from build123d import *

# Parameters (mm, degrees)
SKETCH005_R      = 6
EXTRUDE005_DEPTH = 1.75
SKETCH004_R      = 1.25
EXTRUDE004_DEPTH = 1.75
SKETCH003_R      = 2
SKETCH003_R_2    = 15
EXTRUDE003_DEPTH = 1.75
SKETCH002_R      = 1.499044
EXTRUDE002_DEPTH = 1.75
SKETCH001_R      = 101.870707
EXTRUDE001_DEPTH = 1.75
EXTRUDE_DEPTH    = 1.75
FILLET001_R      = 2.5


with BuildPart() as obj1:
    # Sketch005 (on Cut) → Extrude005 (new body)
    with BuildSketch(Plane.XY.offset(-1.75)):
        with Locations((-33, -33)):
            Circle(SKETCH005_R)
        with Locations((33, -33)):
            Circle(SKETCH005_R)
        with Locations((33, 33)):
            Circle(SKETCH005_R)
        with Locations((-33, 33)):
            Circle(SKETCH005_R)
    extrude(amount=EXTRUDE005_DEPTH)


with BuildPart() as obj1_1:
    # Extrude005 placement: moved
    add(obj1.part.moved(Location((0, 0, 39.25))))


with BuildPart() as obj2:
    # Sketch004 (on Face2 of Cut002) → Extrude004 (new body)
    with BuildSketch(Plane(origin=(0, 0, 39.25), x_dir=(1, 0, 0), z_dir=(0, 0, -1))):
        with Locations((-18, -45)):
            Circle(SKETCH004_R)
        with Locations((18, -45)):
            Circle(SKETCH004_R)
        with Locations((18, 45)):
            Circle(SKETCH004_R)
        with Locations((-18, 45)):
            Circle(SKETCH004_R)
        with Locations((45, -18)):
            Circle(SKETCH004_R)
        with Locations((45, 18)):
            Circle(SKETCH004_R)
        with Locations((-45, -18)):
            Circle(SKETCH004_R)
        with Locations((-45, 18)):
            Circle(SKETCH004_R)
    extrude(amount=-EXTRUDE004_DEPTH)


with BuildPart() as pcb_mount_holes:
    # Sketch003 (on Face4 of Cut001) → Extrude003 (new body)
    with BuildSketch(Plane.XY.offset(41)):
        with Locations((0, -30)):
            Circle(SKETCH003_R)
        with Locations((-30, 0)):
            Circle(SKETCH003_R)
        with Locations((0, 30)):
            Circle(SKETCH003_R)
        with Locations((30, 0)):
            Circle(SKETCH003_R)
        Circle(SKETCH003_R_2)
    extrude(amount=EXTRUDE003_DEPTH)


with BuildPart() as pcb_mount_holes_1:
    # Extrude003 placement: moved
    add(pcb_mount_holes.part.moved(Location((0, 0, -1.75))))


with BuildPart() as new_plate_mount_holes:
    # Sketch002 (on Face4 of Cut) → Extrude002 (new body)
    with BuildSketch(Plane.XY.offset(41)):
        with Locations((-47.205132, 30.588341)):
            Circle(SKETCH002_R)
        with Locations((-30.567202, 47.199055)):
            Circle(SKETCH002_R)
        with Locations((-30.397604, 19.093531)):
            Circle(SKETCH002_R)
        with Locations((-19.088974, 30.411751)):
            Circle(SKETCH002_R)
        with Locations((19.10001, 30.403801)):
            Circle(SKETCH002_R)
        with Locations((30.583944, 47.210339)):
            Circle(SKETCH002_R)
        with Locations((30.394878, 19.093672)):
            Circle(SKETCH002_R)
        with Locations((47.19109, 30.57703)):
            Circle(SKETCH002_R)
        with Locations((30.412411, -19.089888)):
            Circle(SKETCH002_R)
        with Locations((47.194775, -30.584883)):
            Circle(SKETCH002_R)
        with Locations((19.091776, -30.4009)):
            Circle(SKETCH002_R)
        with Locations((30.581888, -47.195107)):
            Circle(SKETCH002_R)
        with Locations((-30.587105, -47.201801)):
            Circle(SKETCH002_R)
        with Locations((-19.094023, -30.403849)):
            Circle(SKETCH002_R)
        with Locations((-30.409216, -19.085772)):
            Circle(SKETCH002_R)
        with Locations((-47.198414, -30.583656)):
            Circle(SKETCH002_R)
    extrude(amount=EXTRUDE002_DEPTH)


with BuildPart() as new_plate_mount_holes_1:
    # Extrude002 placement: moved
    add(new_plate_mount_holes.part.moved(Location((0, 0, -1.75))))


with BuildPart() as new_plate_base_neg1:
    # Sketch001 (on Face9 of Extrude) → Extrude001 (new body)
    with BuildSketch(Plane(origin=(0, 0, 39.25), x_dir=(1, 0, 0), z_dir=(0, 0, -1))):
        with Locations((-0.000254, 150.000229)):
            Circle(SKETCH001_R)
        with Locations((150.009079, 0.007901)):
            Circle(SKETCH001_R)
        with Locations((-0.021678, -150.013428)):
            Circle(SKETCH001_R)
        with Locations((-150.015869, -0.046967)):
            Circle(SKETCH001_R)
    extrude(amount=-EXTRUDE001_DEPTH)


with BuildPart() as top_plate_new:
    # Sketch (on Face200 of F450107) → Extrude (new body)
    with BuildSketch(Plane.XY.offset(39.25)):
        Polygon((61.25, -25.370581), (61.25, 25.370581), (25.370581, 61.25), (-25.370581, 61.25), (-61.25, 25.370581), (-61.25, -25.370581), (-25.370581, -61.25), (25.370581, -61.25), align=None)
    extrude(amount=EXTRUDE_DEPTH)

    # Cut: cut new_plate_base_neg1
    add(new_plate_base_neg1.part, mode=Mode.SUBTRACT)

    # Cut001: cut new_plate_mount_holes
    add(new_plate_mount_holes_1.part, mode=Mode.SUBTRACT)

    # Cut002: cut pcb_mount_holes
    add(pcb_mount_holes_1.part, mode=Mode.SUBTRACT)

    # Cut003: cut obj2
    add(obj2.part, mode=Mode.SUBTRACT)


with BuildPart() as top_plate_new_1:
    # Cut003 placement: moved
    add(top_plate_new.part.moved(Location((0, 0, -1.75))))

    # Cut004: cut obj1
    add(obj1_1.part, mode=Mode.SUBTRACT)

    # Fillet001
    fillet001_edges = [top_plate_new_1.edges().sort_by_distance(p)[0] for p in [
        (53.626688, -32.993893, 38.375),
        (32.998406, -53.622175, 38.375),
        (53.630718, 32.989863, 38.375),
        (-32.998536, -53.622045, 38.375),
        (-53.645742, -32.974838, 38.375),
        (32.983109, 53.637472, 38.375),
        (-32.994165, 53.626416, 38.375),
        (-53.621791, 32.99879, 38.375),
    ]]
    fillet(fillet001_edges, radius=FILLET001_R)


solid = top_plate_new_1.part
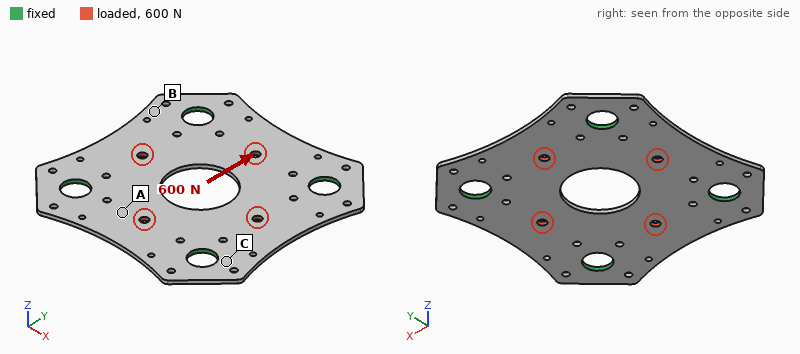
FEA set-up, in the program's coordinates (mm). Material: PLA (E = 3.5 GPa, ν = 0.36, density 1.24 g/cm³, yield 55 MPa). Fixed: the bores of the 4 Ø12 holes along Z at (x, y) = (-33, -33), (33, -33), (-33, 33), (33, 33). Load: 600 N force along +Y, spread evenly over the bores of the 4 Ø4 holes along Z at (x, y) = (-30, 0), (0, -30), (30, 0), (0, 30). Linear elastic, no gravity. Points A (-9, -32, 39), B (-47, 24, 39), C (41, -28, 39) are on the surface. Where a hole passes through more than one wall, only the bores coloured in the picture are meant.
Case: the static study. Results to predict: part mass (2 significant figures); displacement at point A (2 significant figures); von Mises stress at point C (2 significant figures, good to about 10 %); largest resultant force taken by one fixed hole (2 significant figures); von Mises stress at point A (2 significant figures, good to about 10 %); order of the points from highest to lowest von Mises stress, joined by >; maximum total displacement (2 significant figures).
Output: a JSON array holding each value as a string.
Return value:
["18 g", "32 µm", "1.4 MPa", "150 N", "2.3 MPa", "A > C > B", "48 µm"]
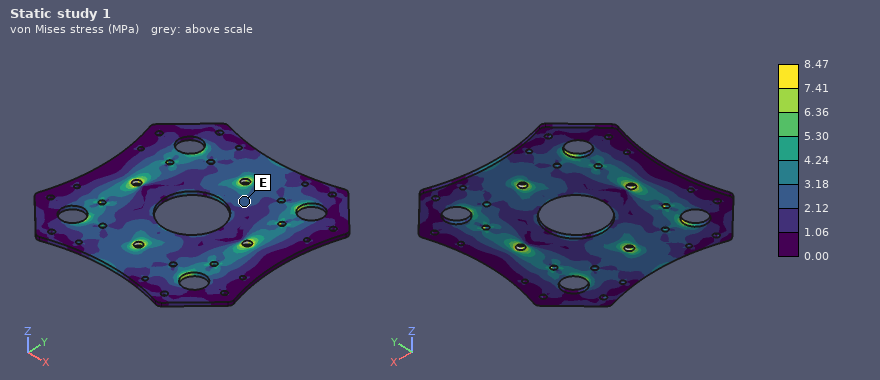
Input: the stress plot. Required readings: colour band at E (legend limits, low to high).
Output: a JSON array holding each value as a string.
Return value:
["2.12 to 3.18 MPa"]
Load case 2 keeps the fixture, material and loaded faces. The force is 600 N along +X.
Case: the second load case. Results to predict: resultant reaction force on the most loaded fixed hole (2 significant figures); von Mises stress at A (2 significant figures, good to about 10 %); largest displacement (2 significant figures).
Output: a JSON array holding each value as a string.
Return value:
["150 N", "3.8 MPa", "48 µm"]
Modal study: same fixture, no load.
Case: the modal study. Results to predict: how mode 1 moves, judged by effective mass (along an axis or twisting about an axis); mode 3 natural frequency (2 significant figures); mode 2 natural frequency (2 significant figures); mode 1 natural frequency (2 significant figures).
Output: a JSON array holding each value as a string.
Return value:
["along Z", "950 Hz", "950 Hz", "740 Hz"]
